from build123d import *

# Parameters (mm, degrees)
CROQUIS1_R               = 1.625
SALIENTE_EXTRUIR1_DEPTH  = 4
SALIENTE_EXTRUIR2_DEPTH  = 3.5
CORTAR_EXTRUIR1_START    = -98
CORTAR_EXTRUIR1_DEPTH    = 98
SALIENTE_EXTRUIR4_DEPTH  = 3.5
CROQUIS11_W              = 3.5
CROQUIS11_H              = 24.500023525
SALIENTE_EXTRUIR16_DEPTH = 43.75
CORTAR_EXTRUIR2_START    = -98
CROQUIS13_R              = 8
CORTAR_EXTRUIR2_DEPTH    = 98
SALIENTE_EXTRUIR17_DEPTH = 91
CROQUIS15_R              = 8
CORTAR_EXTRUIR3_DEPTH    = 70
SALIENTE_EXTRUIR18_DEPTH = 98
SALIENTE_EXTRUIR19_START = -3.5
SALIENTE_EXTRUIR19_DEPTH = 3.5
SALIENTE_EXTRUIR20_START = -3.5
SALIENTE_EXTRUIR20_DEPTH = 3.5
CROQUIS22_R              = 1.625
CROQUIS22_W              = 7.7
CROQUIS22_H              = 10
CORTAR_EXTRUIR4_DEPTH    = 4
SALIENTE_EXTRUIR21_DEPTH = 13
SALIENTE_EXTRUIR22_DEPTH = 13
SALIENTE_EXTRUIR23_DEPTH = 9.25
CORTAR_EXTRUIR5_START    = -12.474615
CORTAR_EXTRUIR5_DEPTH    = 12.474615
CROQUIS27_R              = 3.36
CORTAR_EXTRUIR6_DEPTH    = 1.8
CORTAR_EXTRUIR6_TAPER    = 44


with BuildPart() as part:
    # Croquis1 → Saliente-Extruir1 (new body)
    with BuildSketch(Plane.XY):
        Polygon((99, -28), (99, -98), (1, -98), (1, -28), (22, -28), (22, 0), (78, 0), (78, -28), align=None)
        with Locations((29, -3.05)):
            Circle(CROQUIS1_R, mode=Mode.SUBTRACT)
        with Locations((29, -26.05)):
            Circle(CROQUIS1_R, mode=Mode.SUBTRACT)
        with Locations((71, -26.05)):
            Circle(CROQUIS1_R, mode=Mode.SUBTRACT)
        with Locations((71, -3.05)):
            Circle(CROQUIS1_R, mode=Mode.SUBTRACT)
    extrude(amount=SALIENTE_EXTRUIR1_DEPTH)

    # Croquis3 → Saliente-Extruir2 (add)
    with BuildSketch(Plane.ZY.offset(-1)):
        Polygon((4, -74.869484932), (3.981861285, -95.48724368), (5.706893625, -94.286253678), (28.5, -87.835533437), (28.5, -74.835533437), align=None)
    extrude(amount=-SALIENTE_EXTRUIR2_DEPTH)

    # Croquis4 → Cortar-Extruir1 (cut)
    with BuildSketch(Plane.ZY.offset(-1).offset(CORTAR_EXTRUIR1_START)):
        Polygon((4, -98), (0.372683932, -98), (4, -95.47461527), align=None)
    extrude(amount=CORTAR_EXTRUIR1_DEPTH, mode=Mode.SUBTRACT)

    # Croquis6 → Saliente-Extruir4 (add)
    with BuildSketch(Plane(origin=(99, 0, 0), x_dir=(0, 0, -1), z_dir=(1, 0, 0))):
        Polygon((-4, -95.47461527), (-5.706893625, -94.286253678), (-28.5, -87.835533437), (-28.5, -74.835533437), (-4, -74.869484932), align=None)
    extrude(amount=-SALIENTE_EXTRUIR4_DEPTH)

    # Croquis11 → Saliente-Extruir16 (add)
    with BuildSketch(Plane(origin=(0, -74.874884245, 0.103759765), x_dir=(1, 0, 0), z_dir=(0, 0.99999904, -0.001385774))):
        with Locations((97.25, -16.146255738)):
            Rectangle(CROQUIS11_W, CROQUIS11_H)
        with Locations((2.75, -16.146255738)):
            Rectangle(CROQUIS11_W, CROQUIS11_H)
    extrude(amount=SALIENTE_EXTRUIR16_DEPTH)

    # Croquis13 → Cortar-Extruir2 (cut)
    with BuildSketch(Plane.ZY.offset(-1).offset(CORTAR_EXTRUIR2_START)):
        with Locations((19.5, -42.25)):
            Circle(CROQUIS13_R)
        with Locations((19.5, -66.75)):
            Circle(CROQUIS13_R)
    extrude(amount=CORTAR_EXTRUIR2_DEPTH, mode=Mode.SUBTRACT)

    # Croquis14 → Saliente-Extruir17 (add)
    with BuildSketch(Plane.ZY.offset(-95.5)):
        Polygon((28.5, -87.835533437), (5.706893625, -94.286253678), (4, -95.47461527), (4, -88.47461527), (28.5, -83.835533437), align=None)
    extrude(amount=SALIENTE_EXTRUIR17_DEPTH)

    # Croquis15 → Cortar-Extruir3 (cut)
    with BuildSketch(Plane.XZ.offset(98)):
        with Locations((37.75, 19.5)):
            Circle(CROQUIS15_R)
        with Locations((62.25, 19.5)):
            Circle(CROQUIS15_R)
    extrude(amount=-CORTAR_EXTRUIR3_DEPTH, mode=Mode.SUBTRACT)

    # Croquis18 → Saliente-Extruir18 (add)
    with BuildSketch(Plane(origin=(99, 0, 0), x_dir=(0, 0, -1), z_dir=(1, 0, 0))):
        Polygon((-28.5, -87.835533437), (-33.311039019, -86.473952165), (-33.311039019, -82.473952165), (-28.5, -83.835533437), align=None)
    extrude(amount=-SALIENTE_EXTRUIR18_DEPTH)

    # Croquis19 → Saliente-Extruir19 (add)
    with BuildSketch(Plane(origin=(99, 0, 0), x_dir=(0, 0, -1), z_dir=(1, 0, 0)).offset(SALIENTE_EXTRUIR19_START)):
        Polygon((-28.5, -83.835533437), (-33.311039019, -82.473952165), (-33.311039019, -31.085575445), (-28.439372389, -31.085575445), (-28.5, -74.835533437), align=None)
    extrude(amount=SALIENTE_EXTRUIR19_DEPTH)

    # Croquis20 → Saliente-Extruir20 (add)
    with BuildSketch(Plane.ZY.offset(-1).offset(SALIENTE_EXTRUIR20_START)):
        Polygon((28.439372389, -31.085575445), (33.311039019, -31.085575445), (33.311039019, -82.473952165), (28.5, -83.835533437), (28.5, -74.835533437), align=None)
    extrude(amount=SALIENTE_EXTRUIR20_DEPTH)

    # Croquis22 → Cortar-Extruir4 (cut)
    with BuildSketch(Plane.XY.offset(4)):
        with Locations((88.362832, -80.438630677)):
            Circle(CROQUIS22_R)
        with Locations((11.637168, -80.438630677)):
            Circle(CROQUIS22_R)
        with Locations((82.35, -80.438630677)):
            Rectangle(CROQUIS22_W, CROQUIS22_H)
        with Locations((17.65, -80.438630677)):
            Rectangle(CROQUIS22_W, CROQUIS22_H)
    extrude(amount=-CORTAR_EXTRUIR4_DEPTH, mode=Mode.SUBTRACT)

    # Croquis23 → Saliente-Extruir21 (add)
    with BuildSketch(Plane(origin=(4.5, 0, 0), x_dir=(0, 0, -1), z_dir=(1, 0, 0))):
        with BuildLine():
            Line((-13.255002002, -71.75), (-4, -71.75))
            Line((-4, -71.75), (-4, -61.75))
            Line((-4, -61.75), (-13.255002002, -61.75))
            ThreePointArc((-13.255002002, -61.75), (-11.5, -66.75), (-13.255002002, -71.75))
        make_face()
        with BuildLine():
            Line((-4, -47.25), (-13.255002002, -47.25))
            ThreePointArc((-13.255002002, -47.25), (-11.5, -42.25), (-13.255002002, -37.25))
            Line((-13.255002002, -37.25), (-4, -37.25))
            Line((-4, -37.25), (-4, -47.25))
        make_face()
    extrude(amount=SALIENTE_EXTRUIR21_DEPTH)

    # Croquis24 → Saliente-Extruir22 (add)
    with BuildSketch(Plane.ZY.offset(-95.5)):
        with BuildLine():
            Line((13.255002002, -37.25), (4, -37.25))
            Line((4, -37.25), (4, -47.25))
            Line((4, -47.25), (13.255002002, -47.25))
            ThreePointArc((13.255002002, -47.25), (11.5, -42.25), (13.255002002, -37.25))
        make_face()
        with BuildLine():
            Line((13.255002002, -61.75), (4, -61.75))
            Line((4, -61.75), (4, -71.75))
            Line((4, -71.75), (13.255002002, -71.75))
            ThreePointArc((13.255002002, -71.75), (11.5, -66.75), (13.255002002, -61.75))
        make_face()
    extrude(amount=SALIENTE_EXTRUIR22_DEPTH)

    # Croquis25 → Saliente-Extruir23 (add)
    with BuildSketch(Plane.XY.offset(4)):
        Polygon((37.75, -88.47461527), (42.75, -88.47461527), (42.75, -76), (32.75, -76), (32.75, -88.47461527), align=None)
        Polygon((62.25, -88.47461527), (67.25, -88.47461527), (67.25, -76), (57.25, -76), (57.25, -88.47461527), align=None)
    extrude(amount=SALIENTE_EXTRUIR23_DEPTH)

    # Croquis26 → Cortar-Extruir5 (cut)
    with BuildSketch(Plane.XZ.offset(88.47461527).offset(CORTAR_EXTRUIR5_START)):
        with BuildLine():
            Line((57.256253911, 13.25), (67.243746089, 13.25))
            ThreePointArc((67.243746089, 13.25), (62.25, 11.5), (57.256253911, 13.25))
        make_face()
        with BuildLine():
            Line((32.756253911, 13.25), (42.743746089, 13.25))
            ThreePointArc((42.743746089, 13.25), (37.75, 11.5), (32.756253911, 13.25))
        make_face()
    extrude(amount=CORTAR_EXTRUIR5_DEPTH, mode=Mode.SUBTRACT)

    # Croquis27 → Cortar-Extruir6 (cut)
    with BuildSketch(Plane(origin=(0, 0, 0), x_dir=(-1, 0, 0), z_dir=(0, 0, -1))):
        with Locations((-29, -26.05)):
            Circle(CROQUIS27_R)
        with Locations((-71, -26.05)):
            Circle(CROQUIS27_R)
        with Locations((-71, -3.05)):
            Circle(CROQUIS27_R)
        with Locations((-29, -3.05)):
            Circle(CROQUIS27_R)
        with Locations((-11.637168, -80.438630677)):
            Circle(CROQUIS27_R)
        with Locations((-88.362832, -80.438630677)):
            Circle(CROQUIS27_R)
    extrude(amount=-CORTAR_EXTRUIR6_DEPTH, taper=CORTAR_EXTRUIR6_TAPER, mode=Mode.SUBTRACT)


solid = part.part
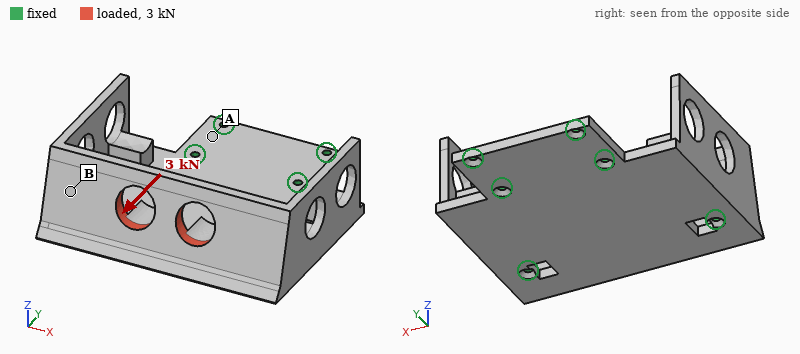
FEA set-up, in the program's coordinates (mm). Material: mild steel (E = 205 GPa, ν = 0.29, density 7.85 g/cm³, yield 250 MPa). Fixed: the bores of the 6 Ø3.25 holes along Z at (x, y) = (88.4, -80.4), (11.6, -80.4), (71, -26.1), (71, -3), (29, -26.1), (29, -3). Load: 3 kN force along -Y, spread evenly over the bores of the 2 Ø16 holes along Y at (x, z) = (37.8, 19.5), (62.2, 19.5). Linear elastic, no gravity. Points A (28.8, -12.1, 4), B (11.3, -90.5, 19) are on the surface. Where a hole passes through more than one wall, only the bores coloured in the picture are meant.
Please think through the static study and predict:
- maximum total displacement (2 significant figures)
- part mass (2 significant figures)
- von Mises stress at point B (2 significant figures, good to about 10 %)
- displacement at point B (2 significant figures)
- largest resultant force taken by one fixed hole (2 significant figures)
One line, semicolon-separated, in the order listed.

0.13 mm; 460 g; 56 MPa; 0.032 mm; 890 N
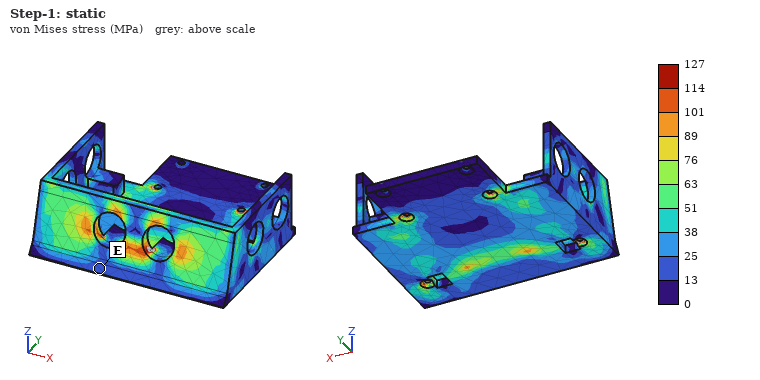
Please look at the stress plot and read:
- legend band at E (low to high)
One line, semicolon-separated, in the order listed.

13 to 25 MPa
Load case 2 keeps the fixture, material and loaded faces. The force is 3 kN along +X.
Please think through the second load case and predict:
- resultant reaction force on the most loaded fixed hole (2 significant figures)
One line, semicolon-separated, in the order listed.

1.5 kN
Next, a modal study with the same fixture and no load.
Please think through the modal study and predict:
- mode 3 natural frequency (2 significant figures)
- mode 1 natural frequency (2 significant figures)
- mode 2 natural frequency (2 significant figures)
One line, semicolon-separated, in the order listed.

3900 Hz; 2400 Hz; 2700 Hz
